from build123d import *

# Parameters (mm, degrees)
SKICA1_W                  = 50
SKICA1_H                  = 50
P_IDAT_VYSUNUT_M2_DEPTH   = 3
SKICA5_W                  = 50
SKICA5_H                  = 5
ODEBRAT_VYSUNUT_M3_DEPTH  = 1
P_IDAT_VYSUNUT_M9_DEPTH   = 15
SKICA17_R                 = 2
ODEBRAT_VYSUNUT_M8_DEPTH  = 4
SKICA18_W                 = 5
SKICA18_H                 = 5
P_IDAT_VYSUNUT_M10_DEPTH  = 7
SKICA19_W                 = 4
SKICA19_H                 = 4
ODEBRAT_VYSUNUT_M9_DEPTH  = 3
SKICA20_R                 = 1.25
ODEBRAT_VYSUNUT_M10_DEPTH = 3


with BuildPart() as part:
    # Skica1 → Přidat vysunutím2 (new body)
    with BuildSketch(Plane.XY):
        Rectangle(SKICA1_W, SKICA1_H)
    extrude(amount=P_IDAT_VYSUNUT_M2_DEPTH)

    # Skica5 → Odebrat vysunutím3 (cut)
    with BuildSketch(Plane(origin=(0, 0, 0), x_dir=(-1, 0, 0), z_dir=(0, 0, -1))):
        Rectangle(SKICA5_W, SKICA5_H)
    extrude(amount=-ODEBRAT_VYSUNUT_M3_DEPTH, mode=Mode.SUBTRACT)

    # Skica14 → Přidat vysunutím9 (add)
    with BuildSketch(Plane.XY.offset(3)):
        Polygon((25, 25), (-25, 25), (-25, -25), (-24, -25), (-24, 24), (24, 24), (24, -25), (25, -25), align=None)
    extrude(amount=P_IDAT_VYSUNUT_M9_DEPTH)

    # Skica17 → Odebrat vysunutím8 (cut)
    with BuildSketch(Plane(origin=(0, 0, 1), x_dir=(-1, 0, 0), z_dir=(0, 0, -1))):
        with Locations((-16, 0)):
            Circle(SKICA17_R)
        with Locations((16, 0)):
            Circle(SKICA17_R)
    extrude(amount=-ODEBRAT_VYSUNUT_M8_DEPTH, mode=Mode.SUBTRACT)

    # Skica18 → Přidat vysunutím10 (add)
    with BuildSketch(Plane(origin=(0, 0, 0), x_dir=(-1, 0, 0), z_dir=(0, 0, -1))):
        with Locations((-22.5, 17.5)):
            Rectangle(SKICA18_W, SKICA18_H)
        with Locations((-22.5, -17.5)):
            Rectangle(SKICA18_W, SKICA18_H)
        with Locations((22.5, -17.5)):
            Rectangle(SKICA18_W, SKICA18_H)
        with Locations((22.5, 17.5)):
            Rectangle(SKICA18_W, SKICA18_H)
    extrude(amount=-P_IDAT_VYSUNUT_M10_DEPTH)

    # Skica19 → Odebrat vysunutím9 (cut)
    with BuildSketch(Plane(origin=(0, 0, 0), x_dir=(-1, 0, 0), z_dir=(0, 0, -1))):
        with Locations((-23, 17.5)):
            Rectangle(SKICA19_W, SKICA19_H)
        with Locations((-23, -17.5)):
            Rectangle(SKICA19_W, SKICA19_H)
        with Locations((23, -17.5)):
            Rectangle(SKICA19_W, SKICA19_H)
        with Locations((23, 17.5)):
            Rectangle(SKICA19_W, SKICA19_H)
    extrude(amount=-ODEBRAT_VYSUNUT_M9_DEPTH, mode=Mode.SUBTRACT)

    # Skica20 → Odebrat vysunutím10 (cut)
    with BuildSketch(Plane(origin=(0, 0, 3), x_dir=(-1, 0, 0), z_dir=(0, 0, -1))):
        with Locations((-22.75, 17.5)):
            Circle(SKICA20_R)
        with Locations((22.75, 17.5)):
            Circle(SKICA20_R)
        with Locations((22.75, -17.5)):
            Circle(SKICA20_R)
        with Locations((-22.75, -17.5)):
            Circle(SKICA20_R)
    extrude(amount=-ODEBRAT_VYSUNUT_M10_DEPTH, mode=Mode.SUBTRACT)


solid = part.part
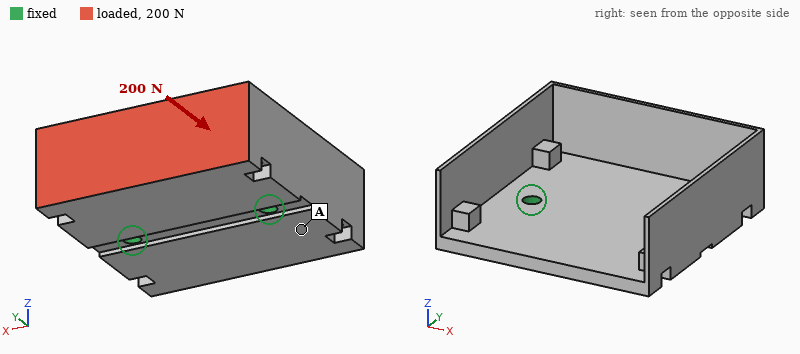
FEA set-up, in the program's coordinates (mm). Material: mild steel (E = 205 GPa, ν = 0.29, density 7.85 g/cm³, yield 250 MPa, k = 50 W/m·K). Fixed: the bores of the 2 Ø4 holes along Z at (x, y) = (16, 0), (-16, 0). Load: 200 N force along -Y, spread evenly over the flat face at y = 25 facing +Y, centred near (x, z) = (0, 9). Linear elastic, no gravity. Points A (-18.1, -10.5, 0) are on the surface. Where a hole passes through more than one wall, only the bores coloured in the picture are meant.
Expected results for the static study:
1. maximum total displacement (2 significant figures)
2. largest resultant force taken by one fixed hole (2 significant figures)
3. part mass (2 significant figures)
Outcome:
67 µm
100 N
74 g
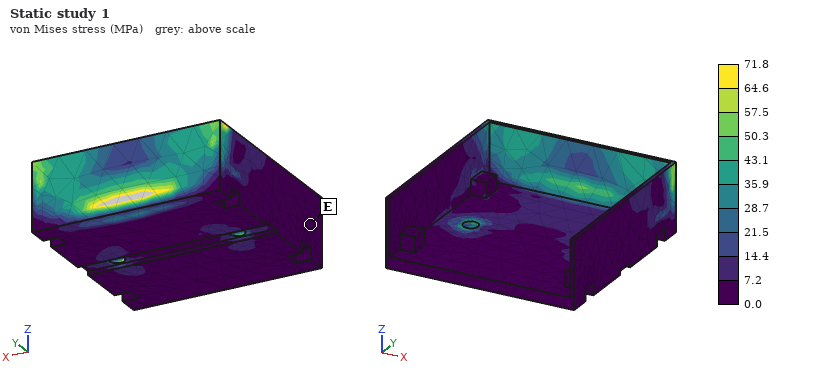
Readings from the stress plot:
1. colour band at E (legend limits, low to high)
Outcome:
0.0 to 7.2 MPa
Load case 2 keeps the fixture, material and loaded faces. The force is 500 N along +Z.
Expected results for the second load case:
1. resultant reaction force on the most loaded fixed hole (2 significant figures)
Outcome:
250 N
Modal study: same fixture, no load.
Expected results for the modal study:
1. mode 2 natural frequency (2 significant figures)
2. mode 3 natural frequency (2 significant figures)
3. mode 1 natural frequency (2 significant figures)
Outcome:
3300 Hz
4200 Hz
2200 Hz
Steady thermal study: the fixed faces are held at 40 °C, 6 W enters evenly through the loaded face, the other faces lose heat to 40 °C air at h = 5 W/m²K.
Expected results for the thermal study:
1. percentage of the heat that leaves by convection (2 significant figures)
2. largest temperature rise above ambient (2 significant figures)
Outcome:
7.7 %
33 K
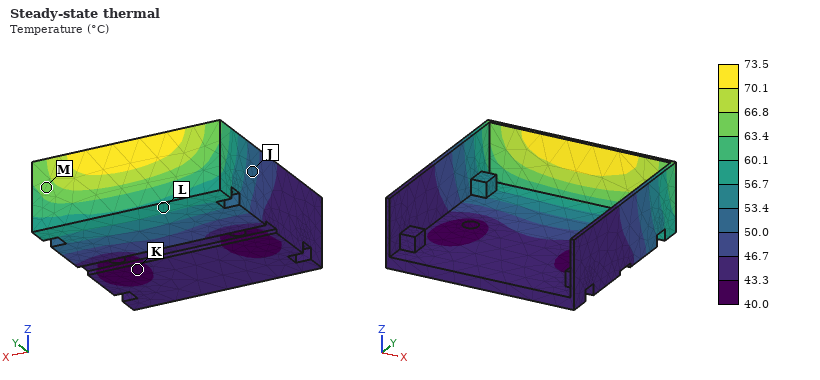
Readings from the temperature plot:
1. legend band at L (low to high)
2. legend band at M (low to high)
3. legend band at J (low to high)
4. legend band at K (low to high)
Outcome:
56.7 to 60.1 °C
63.4 to 66.8 °C
50.0 to 53.4 °C
40.0 to 43.3 °C
